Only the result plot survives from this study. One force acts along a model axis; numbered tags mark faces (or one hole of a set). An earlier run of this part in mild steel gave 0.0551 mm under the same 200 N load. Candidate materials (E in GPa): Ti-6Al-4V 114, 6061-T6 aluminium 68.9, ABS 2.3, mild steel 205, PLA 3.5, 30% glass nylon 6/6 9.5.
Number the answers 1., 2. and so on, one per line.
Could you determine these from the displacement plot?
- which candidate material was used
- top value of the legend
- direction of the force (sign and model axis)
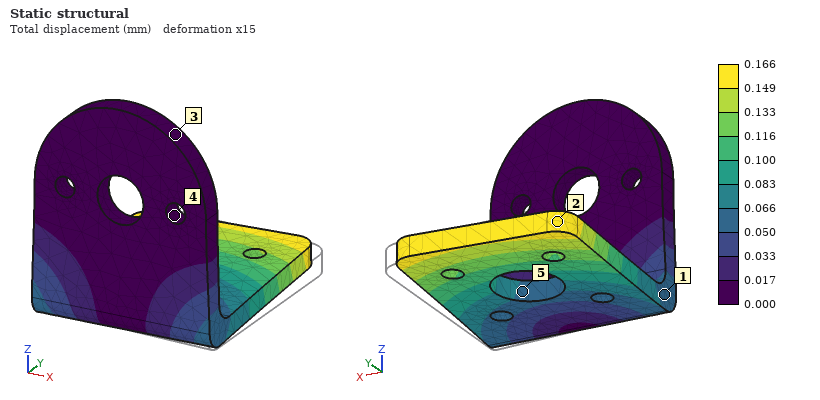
1. 6061-T6 aluminium
2. 0.166 mm
3. -X
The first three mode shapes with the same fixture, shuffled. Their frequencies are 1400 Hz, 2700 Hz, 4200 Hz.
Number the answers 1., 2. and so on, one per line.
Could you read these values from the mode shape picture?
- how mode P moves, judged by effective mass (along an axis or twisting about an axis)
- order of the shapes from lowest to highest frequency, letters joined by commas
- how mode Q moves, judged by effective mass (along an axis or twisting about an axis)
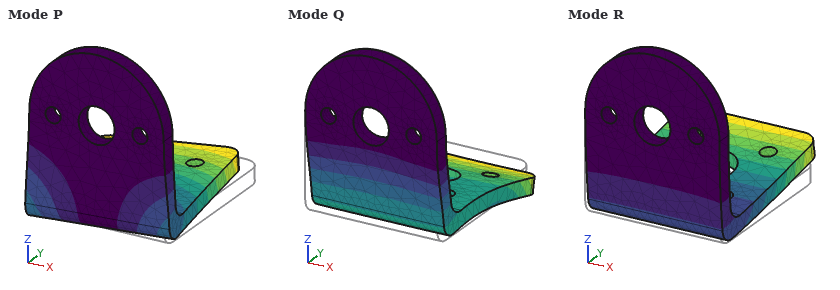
1. along X
2. R, P, Q
3. along Y
